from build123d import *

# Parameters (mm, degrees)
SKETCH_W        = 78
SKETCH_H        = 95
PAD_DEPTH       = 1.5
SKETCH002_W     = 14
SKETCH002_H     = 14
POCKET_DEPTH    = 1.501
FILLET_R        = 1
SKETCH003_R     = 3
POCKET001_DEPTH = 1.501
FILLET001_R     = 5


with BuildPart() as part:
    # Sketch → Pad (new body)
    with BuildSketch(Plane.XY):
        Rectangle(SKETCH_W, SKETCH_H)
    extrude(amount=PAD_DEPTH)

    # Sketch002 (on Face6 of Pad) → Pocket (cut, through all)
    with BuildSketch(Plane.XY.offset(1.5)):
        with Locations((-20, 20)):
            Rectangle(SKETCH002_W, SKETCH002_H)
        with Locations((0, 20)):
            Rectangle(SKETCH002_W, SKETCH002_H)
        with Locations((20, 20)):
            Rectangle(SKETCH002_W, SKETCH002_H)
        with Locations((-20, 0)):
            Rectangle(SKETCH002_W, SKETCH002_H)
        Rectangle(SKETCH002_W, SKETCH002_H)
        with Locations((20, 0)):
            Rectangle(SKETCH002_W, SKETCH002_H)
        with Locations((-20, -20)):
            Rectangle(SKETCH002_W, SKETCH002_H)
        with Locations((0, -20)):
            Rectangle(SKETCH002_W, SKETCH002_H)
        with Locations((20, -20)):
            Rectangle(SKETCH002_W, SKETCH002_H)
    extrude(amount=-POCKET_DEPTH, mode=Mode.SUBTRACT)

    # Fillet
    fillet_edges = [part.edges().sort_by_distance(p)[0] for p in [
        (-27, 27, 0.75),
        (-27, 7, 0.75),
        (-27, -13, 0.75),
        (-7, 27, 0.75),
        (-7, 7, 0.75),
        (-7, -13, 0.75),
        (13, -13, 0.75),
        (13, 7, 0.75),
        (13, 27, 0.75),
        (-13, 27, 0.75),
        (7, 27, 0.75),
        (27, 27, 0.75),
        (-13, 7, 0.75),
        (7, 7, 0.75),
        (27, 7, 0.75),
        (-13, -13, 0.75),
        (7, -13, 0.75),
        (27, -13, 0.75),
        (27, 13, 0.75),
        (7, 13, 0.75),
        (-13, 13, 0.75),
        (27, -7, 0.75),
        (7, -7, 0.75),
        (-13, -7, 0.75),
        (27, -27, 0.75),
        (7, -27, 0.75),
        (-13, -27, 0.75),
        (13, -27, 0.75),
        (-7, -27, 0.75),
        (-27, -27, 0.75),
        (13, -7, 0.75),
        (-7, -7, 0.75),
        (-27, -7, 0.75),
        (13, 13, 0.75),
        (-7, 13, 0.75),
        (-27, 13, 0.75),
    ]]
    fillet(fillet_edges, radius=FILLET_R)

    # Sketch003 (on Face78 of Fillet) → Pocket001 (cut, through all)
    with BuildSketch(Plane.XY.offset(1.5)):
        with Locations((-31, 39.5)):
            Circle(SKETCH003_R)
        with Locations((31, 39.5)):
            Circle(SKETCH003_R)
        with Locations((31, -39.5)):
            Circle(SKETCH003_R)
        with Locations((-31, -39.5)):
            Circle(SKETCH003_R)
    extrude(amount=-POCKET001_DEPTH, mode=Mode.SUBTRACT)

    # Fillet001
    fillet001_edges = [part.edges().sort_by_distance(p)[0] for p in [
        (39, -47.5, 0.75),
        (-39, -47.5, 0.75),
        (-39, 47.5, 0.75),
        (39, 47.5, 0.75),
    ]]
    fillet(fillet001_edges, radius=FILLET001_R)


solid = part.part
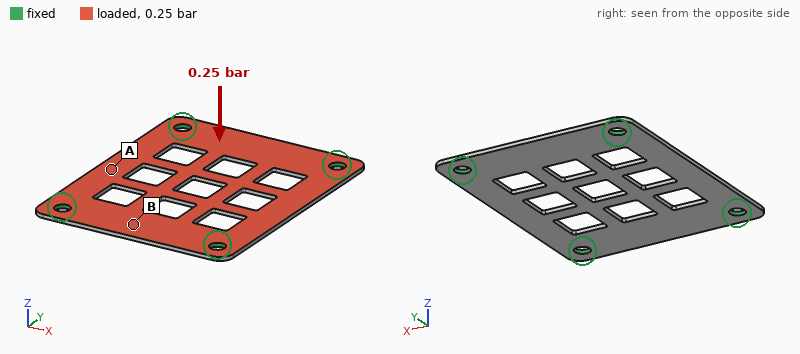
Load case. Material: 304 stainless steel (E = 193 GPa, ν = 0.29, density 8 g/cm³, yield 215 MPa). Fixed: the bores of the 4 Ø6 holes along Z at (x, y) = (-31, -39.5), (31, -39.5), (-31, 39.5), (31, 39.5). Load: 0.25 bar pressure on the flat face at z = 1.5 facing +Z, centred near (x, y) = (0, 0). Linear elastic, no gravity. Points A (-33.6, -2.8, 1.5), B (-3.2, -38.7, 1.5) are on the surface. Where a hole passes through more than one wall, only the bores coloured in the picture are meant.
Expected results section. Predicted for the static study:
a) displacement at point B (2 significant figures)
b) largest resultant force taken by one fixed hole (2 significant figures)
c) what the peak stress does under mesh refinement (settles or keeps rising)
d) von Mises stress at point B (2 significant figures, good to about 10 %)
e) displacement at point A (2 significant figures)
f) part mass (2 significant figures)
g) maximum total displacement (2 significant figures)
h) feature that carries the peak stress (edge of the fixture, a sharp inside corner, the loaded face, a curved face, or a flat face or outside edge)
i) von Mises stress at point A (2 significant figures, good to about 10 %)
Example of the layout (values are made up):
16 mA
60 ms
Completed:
18 µm
34 N
keeps rising
12 MPa
43 µm
66 g
65 µm
edge of the fixture
19 MPa
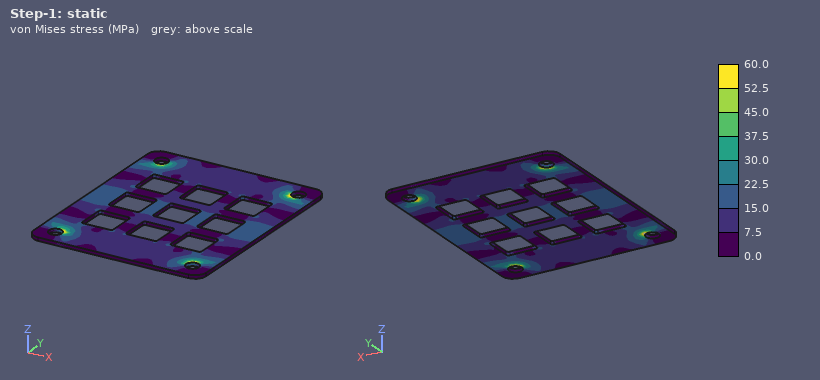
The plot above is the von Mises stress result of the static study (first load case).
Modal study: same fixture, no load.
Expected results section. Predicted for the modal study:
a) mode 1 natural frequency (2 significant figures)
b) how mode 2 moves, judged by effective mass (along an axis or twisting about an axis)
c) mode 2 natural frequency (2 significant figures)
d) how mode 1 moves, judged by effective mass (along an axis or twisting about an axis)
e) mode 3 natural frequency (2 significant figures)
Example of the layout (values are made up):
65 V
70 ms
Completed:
1100 Hz
twisting about Y
1500 Hz
along Z
1900 Hz
